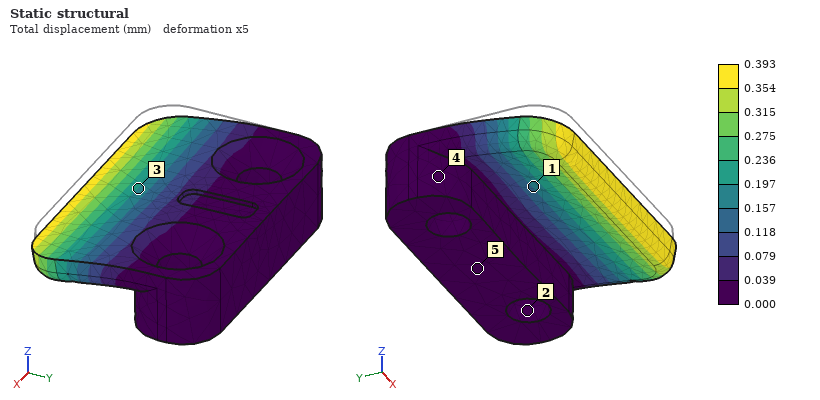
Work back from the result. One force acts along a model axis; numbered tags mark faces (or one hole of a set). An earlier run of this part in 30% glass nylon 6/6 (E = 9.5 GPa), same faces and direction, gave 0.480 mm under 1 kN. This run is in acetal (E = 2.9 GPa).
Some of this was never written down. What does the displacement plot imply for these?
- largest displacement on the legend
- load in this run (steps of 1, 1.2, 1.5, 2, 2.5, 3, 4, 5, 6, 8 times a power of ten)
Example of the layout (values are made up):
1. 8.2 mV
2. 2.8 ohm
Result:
1. 0.393 mm
2. 250 N
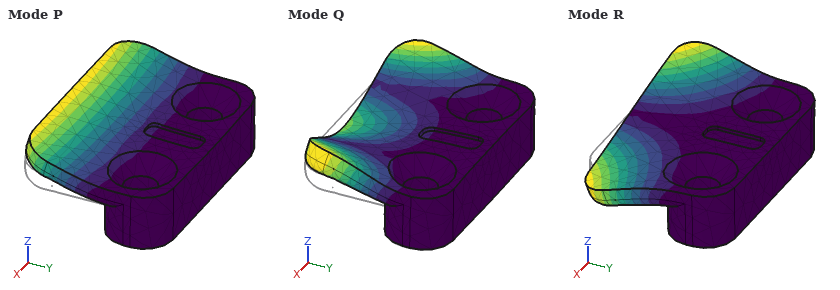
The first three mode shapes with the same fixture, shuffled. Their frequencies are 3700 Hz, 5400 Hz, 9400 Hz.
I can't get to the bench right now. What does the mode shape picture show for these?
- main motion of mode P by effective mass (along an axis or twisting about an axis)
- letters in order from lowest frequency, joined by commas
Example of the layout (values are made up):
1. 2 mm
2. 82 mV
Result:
1. along Z
2. P, R, Q
